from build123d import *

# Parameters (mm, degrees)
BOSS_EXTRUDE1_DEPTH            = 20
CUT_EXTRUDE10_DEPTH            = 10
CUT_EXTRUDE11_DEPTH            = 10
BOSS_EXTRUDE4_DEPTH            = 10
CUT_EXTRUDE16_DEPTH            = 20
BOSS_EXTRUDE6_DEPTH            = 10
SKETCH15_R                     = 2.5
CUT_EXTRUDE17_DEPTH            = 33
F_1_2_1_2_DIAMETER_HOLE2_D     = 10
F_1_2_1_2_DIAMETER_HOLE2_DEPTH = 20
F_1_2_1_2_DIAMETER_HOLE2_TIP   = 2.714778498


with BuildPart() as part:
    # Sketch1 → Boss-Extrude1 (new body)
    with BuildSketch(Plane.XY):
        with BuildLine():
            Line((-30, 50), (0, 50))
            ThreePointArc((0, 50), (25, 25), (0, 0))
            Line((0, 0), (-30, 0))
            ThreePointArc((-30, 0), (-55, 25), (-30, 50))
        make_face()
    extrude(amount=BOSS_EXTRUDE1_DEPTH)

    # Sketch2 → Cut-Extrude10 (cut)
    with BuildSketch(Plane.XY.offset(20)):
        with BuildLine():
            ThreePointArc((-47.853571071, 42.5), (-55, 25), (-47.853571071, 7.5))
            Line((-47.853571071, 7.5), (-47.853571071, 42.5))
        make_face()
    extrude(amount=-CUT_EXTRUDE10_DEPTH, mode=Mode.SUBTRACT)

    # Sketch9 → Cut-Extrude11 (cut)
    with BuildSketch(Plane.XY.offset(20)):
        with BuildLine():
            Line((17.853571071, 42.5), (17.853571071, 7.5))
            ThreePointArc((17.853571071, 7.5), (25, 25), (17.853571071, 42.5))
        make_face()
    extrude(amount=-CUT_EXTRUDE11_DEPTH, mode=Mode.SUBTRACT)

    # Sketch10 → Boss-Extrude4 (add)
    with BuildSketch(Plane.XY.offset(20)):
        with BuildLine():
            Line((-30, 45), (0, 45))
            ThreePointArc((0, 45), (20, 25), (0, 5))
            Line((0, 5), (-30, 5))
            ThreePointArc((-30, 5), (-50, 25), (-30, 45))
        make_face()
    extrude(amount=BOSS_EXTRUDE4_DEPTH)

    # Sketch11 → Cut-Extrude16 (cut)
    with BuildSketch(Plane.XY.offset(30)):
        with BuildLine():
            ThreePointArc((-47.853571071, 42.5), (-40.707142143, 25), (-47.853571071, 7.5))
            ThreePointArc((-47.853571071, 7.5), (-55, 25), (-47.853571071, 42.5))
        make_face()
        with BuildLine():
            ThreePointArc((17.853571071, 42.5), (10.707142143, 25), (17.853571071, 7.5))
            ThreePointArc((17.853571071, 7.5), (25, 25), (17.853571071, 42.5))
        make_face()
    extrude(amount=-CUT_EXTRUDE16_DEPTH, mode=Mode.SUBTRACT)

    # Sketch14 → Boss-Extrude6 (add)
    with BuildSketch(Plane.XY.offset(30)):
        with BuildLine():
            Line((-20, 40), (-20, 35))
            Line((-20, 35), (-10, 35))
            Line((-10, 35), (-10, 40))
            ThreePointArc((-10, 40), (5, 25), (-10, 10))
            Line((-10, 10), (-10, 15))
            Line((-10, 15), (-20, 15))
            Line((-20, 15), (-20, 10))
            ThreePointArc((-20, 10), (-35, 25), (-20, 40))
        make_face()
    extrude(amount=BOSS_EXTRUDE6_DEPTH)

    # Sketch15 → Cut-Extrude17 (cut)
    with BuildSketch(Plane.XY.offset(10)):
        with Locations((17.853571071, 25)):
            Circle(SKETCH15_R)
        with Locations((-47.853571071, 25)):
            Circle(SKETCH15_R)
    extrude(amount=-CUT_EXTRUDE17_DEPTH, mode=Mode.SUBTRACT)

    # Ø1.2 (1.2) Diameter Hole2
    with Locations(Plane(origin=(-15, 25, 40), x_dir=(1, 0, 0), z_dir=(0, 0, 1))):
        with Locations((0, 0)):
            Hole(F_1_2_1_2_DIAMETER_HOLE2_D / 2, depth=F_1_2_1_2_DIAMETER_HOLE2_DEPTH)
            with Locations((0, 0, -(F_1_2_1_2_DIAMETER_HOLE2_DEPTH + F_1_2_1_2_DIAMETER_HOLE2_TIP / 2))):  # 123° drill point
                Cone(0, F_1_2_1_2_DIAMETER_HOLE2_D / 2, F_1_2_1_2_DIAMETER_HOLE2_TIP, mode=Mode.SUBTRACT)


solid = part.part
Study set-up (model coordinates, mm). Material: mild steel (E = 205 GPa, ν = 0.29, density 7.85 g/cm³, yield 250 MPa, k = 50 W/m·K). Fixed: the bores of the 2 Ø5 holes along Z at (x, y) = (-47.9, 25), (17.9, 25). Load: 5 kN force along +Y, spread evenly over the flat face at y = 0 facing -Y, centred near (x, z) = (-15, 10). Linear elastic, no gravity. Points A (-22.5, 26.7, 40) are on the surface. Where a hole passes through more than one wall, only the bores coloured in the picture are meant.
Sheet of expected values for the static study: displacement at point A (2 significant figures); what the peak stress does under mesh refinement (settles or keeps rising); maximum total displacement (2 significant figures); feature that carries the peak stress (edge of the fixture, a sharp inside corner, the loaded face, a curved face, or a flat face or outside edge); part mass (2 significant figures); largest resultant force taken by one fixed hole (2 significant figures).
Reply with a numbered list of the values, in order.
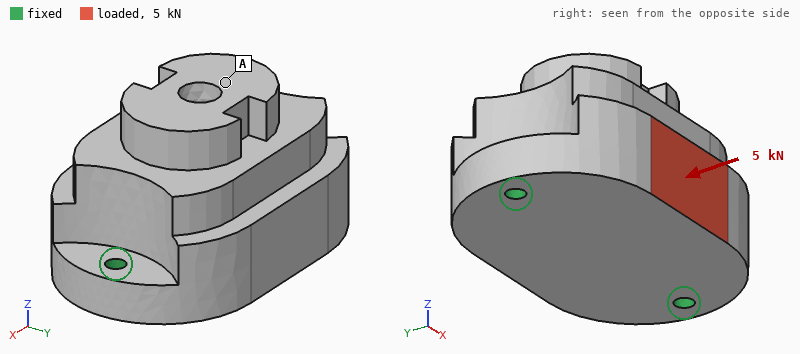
1. 8.8 µm
2. keeps rising
3. 9.4 µm
4. edge of the fixture
5. 710 g
6. 2.5 kN
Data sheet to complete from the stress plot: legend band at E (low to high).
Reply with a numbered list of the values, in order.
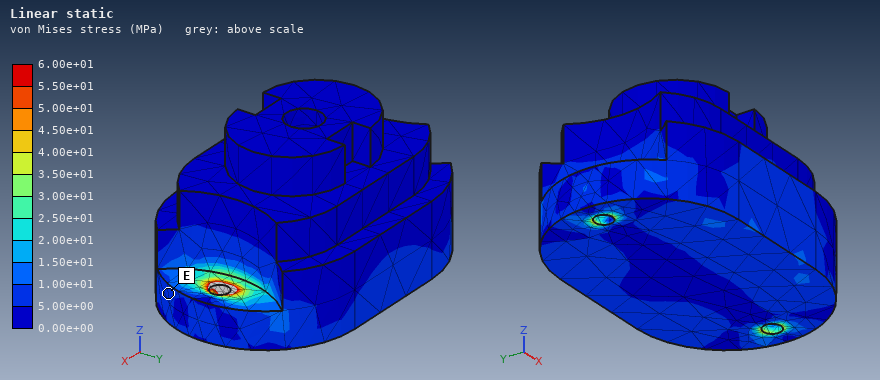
1. 5.00e+00 to 1.00e+01 MPa
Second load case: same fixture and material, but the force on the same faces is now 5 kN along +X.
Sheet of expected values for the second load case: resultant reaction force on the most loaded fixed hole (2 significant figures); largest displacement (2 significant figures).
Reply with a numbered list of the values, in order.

1. 3.1 kN
2. 2.9 µm
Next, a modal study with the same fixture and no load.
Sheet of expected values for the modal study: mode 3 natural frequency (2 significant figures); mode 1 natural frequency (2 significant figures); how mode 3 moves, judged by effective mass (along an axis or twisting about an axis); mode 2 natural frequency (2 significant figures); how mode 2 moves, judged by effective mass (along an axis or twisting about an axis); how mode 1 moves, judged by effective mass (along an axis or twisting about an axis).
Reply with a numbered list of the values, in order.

1. 11 kHz
2. 3400 Hz
3. along X
4. 8300 Hz
5. along Z
6. along Y
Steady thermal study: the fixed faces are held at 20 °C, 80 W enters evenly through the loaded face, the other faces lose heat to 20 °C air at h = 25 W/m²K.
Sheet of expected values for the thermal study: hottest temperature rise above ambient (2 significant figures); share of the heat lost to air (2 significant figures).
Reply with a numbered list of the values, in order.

1. 72 K
2. 14 %
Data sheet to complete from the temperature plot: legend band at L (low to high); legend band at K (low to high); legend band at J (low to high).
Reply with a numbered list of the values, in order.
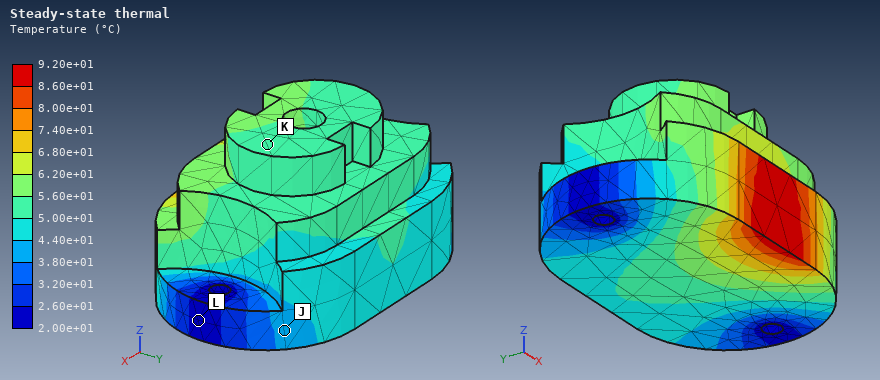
1. 2.00e+01 to 2.60e+01 °C
2. 5.00e+01 to 5.60e+01 °C
3. 3.80e+01 to 4.40e+01 °C
